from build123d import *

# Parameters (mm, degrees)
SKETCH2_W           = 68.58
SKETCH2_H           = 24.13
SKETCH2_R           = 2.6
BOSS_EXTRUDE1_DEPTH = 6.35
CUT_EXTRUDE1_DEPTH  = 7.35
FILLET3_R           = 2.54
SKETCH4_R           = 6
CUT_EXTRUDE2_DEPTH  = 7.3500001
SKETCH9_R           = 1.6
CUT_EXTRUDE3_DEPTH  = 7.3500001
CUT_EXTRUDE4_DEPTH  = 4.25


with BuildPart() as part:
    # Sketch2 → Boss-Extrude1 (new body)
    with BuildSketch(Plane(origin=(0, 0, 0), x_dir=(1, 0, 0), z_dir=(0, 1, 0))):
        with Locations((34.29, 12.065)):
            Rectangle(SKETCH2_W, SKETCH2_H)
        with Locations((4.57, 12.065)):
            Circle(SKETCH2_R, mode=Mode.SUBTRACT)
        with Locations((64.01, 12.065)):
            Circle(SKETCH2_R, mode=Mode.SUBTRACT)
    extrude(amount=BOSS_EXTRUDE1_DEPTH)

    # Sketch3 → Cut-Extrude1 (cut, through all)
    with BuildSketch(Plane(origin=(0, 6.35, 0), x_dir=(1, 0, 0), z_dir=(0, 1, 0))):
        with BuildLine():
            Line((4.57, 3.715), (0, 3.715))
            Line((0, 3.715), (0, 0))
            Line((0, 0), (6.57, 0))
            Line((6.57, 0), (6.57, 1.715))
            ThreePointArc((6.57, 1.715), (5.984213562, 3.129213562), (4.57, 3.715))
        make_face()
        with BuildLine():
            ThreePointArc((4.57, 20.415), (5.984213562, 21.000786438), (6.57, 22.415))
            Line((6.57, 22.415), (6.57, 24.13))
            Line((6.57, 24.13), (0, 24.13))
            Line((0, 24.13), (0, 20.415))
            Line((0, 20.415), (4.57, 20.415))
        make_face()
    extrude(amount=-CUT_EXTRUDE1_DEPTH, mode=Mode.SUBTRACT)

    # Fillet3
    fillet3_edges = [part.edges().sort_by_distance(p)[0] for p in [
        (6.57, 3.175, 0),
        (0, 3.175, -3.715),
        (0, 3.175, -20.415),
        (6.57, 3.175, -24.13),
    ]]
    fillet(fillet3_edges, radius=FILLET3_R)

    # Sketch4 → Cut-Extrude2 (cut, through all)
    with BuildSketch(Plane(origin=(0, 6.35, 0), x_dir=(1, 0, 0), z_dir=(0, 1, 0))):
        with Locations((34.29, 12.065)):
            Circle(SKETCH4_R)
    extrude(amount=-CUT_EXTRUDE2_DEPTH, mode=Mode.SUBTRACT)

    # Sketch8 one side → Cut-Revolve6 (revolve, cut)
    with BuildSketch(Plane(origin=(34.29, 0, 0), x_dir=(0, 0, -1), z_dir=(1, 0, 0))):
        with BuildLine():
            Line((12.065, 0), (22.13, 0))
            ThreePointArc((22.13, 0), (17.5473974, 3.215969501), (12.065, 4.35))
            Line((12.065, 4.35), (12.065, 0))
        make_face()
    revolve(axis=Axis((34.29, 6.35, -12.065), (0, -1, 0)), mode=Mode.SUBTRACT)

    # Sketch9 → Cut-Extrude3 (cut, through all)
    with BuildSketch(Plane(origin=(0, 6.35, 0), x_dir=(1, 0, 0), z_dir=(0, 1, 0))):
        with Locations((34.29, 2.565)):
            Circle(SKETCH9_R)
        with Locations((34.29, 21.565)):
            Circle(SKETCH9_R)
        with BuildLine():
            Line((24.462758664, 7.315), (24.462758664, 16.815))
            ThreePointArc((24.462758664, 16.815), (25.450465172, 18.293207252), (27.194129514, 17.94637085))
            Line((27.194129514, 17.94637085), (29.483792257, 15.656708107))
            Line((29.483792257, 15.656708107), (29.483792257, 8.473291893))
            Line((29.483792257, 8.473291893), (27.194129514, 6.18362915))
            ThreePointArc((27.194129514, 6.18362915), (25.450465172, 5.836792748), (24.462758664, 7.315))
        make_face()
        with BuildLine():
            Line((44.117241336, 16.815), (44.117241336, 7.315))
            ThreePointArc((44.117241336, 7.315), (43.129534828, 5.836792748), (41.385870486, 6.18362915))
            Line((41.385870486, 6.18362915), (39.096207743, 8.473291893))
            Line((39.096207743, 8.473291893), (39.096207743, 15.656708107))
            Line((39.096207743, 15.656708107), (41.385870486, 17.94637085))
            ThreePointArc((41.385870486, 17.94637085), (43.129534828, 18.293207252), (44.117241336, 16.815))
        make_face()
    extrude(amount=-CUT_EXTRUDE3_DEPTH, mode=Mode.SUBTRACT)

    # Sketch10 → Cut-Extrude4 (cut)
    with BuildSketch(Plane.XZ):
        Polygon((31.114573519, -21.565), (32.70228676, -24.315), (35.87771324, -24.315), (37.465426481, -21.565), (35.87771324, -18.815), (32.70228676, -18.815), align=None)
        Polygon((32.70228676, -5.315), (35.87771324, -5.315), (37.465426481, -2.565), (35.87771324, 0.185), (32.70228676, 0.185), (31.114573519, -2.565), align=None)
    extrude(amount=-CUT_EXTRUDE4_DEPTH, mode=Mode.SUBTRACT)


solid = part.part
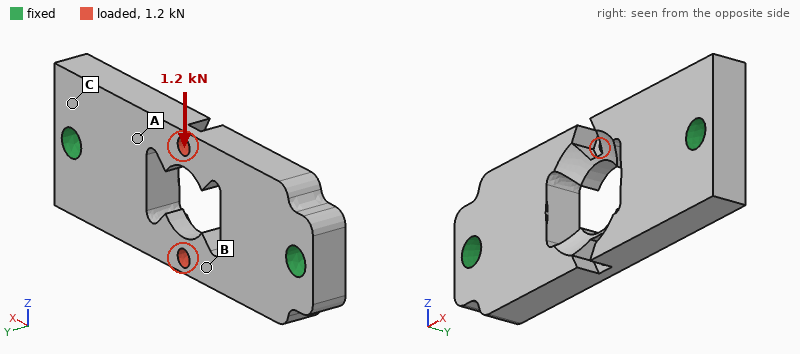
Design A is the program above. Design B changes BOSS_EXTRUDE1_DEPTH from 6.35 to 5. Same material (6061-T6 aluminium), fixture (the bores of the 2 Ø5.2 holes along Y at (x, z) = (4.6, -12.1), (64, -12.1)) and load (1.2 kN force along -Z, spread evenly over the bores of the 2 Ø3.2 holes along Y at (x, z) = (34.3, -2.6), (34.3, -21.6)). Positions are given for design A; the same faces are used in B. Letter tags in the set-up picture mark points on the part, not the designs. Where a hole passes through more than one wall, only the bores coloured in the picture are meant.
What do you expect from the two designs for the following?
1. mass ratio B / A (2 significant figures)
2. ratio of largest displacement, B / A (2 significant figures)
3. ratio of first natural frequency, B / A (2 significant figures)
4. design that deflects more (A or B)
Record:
0.78
1.7
0.84
B
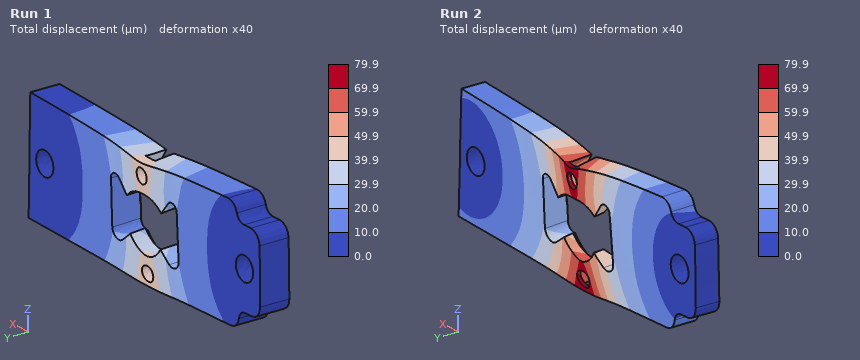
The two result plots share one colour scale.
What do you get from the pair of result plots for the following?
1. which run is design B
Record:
Run 2
